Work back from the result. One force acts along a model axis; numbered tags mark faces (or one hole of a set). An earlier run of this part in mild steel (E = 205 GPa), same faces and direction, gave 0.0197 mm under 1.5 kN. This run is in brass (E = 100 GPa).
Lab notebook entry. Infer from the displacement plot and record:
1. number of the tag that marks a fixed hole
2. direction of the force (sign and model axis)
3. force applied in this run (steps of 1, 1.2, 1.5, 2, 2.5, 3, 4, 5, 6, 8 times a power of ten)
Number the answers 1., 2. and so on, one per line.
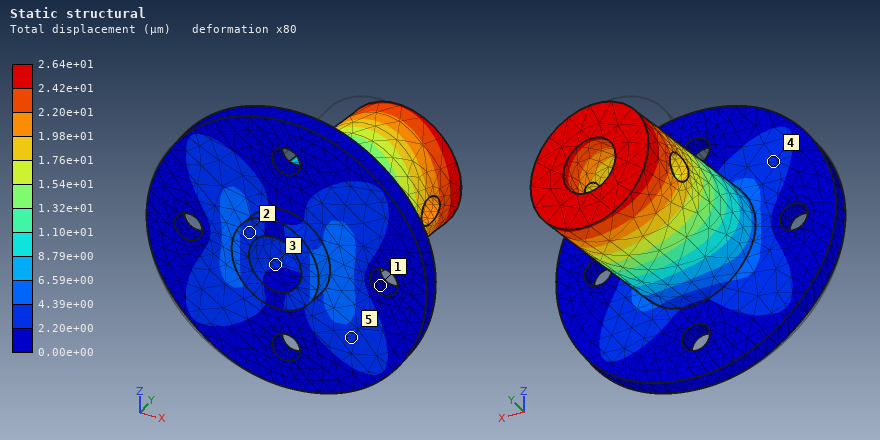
1. 1
2. +X
3. 1 kN
